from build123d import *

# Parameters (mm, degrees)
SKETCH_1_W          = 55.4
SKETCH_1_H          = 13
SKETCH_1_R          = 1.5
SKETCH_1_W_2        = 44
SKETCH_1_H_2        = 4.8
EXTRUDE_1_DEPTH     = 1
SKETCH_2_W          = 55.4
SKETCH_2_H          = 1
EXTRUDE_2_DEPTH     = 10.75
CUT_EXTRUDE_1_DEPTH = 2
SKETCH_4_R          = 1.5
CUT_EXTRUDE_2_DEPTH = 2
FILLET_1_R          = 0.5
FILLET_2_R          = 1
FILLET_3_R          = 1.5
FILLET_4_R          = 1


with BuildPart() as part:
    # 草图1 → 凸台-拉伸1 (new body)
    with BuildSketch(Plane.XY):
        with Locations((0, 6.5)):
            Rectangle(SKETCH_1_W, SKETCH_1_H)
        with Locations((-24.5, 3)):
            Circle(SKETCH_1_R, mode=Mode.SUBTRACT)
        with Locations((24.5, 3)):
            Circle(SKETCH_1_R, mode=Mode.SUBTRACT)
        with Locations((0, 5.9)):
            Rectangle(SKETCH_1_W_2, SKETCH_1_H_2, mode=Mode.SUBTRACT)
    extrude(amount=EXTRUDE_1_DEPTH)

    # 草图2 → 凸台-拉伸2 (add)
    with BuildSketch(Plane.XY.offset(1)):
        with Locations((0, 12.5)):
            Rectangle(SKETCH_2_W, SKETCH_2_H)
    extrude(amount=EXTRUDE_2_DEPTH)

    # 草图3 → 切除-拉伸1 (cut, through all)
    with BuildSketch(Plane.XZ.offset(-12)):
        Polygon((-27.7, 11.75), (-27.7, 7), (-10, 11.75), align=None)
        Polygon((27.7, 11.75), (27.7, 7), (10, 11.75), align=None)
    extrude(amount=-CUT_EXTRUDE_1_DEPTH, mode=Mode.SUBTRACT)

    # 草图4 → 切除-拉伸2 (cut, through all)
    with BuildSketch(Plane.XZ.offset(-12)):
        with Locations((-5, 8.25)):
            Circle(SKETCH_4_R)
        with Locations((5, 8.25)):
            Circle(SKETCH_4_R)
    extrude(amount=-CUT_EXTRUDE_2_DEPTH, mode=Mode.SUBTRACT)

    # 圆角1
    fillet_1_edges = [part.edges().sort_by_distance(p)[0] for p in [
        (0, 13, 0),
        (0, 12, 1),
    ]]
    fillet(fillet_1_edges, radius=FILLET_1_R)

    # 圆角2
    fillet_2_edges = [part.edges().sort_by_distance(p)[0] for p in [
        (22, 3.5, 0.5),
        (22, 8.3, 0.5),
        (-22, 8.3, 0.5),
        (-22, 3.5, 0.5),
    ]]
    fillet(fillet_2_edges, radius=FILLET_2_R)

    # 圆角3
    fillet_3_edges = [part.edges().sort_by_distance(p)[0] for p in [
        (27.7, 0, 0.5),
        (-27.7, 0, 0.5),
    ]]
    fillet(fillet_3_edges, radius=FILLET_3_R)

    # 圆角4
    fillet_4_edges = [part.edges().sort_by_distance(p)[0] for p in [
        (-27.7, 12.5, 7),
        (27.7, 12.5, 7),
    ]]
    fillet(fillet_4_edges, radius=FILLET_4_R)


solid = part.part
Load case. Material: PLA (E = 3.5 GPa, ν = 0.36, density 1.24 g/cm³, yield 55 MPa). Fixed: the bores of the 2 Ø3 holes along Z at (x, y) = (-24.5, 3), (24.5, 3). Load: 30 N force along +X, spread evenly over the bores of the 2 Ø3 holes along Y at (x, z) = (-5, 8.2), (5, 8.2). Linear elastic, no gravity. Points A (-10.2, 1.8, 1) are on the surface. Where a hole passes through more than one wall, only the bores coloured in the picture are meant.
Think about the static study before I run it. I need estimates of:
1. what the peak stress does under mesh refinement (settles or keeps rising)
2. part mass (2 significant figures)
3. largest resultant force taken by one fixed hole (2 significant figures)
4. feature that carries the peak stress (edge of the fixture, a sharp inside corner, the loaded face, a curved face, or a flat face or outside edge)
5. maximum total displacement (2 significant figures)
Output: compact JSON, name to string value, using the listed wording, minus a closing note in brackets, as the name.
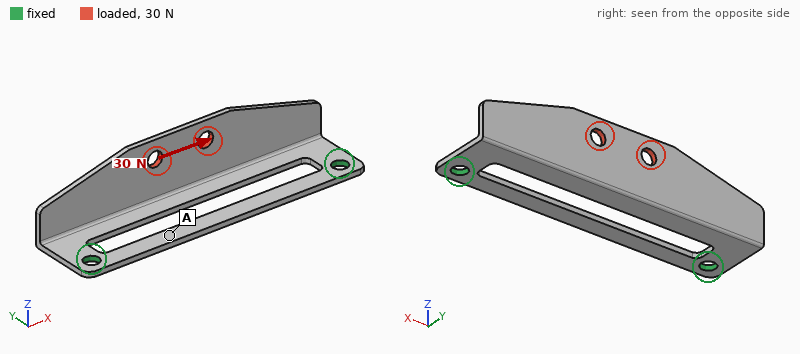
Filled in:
{"what the peak stress does under mesh refinement": "keeps rising", "part mass": "1.2 g", "largest resultant force taken by one fixed hole": "16 N", "feature that carries the peak stress": "edge of the fixture", "maximum total displacement": "0.46 mm"}
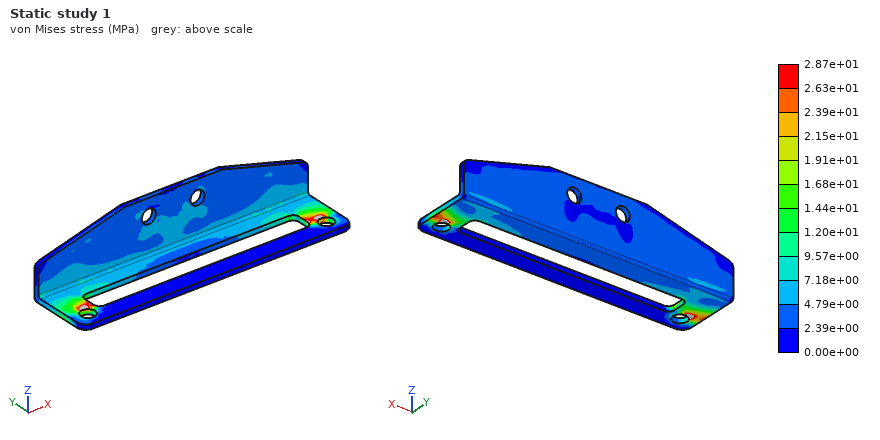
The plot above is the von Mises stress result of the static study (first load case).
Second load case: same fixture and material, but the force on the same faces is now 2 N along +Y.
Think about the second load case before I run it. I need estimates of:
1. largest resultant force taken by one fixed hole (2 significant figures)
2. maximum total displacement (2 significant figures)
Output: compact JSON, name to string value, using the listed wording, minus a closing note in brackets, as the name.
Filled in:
{"largest resultant force taken by one fixed hole": "1.7 N", "maximum total displacement": "0.63 mm"}
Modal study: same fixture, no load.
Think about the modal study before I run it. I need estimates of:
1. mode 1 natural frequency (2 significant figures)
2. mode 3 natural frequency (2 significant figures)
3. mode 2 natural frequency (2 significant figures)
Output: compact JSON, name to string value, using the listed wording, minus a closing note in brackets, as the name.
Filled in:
{"mode 1 natural frequency": "530 Hz", "mode 3 natural frequency": "1300 Hz", "mode 2 natural frequency": "810 Hz"}
